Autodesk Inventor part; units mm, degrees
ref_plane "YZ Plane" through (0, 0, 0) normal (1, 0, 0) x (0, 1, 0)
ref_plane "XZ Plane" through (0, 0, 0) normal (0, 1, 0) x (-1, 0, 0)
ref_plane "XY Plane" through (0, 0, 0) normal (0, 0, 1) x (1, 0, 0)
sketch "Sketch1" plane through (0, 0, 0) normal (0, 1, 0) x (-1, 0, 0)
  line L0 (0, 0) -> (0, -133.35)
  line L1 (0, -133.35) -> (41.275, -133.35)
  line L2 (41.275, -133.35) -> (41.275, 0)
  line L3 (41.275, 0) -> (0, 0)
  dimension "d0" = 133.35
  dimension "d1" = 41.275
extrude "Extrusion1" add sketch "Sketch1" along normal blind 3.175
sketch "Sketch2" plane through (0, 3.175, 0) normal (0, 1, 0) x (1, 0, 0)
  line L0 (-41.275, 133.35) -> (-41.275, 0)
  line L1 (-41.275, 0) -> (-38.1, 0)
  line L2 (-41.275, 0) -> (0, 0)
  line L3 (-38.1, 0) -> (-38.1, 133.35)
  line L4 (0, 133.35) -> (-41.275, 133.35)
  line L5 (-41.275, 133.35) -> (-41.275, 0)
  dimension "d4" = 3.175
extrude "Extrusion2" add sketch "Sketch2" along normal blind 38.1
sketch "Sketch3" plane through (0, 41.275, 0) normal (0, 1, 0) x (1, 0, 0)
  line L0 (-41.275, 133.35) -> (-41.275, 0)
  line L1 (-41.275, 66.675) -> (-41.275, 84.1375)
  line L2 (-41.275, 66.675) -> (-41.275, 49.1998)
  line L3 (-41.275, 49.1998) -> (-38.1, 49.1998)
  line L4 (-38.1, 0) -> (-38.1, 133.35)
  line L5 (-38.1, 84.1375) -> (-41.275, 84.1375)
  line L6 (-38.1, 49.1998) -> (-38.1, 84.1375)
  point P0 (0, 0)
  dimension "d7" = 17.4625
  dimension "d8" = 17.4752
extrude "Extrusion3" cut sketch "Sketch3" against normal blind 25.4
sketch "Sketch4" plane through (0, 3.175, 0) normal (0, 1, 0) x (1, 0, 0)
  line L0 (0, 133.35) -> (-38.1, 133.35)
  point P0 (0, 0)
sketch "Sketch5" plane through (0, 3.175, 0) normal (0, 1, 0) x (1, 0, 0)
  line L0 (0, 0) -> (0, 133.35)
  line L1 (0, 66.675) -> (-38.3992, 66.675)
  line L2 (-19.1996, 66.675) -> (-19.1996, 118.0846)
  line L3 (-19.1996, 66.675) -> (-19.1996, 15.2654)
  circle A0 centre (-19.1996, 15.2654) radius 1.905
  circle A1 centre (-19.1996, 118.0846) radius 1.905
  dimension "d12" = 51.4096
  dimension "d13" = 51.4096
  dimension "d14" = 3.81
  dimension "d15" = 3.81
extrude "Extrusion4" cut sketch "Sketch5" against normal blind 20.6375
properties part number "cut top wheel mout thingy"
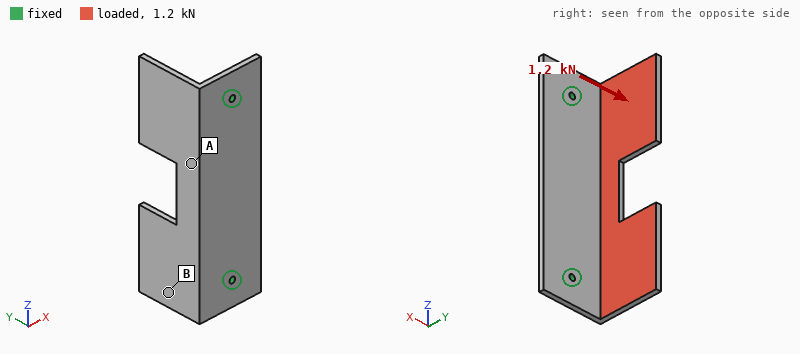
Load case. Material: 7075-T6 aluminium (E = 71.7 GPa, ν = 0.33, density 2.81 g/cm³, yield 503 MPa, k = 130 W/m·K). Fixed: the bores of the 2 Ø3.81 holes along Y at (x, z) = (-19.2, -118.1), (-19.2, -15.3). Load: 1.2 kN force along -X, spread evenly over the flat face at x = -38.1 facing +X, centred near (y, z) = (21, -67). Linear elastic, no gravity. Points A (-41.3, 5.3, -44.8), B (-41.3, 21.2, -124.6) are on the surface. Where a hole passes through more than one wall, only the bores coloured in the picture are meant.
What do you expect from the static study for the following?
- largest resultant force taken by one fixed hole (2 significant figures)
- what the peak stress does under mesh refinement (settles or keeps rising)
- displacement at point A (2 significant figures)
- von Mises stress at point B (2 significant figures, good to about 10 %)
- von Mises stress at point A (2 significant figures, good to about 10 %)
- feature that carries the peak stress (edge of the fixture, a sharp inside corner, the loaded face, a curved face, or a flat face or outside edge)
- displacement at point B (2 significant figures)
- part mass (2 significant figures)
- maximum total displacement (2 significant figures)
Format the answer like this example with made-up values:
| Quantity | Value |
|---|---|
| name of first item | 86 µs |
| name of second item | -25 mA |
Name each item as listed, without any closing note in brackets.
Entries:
| Quantity | Value |
|---|---|
| largest resultant force taken by one fixed hole | 600 N |
| what the peak stress does under mesh refinement | keeps rising |
| displacement at point A | 0.42 mm |
| von Mises stress at point B | 30 MPa |
| von Mises stress at point A | 71 MPa |
| feature that carries the peak stress | edge of the fixture |
| displacement at point B | 0.77 mm |
| part mass | 86 g |
| maximum total displacement | 1.5 mm |
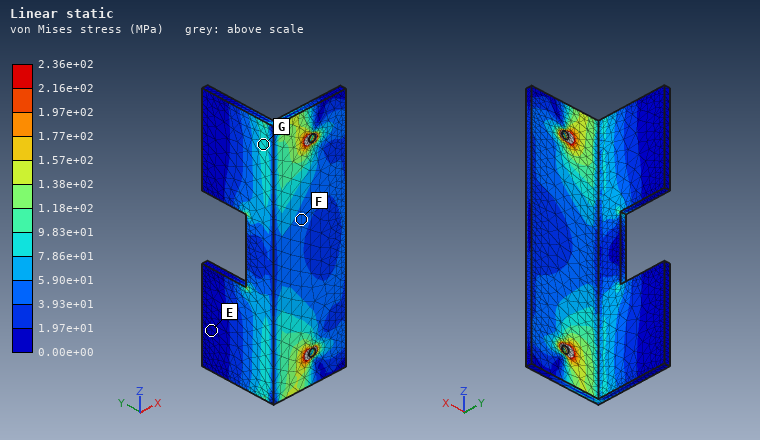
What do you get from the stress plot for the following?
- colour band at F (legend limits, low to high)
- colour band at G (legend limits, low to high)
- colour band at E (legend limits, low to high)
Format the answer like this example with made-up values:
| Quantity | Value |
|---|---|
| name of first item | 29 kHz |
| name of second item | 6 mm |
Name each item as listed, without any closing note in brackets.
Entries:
| Quantity | Value |
|---|---|
| colour band at F | 3.93e+01 to 5.90e+01 MPa |
| colour band at G | 7.86e+01 to 9.83e+01 MPa |
| colour band at E | 0.00e+00 to 1.97e+01 MPa |
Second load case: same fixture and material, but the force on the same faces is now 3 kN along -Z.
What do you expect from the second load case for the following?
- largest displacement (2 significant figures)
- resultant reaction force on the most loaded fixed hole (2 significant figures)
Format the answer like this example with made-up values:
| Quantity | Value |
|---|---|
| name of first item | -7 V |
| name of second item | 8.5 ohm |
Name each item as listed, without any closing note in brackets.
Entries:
| Quantity | Value |
|---|---|
| largest displacement | 0.65 mm |
| resultant reaction force on the most loaded fixed hole | 1.7 kN |
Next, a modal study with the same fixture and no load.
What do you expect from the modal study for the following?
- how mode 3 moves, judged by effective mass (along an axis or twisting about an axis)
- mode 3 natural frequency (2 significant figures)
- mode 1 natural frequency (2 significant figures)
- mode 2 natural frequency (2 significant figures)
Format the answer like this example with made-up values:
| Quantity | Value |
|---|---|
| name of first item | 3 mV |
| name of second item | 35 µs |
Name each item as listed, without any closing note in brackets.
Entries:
| Quantity | Value |
|---|---|
| how mode 3 moves, judged by effective mass | along Y |
| mode 3 natural frequency | 1800 Hz |
| mode 1 natural frequency | 820 Hz |
| mode 2 natural frequency | 1100 Hz |
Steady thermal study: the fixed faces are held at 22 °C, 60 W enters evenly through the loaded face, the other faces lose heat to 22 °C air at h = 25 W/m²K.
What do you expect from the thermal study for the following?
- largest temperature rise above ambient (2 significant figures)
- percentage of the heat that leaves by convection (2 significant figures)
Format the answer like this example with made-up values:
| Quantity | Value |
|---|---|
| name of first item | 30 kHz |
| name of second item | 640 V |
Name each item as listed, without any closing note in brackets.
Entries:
| Quantity | Value |
|---|---|
| largest temperature rise above ambient | 59 K |
| percentage of the heat that leaves by convection | 23 % |
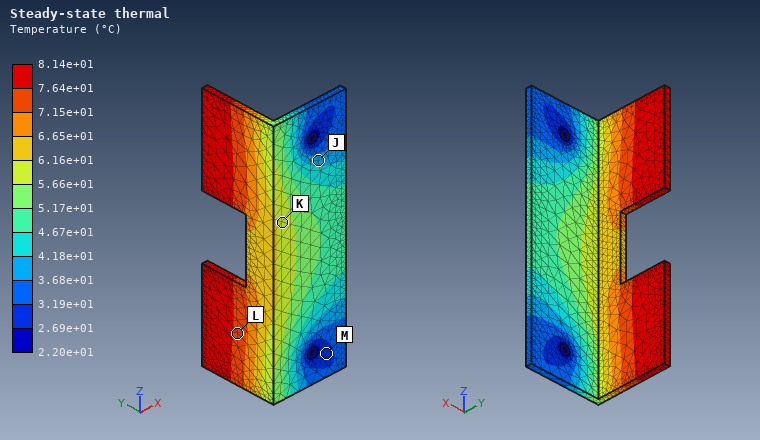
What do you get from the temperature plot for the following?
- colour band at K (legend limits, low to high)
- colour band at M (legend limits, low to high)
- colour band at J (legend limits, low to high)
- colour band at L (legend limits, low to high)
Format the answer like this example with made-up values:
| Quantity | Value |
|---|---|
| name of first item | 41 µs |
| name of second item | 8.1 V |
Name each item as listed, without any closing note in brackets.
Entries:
| Quantity | Value |
|---|---|
| colour band at K | 5.66e+01 to 6.16e+01 °C |
| colour band at M | 2.69e+01 to 3.19e+01 °C |
| colour band at J | 3.68e+01 to 4.18e+01 °C |
| colour band at L | 7.15e+01 to 7.64e+01 °C |
